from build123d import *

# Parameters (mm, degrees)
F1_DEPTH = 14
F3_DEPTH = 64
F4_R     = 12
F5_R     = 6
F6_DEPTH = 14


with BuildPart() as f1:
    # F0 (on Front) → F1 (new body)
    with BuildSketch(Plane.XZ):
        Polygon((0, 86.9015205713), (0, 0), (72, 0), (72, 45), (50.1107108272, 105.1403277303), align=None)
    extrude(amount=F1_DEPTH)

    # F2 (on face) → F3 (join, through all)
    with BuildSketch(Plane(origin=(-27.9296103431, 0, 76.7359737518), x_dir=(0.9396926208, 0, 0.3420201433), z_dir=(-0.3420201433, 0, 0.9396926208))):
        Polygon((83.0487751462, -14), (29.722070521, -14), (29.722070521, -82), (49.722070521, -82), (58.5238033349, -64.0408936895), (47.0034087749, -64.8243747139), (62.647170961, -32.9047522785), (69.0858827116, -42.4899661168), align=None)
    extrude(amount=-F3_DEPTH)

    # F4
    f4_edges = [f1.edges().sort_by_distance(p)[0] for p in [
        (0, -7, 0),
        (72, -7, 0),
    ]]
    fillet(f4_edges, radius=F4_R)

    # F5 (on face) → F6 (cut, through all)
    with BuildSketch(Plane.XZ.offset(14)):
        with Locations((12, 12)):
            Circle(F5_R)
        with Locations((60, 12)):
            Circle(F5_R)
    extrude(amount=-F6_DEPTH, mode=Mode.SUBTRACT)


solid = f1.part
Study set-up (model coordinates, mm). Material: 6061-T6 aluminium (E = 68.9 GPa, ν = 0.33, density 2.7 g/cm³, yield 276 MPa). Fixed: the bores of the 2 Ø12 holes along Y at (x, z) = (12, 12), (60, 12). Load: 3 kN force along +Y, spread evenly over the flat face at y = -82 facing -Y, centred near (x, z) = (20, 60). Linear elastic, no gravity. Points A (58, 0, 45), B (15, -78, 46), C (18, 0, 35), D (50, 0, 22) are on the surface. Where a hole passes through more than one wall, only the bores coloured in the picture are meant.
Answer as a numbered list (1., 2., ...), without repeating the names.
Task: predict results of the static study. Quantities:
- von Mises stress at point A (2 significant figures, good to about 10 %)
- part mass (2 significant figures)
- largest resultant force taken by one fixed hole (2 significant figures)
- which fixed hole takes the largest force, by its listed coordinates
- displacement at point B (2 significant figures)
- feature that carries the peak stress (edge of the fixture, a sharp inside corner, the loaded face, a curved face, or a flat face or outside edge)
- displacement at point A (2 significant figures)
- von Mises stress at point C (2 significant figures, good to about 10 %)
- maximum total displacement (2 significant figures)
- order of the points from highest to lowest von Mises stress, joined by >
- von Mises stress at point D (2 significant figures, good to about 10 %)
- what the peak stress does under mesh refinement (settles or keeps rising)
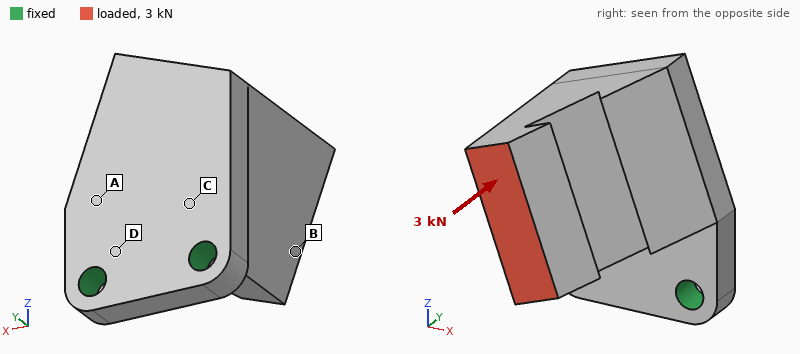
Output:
1. 16 MPa
2. 610 g
3. 2.4 kN
4. (12, 12)
5. 0.18 mm
6. edge of the fixture
7. 0.046 mm
8. 26 MPa
9. 0.25 mm
10. D > C > A > B
11. 36 MPa
12. keeps rising
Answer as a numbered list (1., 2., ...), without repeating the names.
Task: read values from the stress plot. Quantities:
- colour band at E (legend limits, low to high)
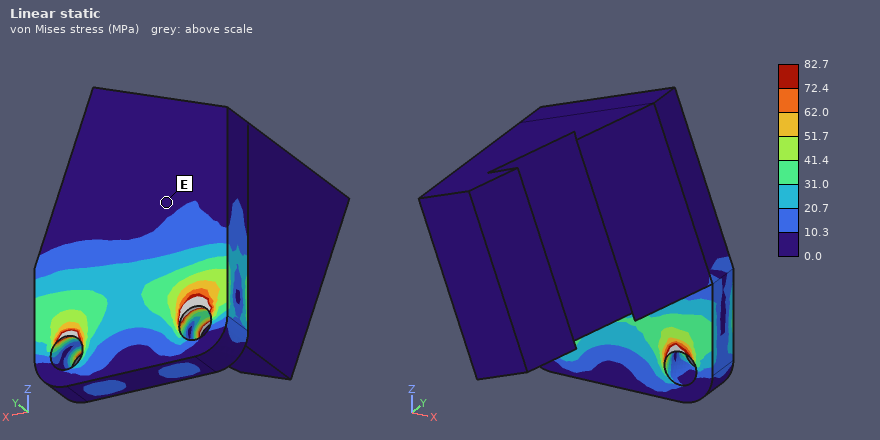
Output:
1. 0.0 to 10.3 MPa
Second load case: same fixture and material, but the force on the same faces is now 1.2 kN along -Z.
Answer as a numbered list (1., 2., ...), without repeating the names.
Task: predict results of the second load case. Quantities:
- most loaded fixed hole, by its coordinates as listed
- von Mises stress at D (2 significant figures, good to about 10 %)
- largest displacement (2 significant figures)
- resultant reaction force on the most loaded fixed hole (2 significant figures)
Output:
1. (12, 12)
2. 29 MPa
3. 0.22 mm
4. 1.0 kN
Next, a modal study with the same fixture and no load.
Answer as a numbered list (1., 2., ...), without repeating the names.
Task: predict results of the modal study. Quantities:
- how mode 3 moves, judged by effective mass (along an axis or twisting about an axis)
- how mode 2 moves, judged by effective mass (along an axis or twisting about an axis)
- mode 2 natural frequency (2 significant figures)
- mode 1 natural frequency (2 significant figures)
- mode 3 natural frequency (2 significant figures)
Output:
1. along X
2. along X
3. 2100 Hz
4. 840 Hz
5. 4600 Hz
